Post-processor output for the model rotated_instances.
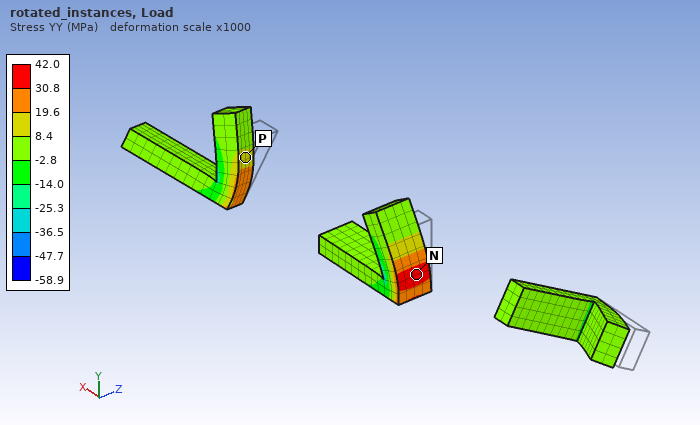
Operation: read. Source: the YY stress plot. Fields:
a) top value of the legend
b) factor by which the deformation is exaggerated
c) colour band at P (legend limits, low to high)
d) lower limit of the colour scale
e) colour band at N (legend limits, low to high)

42.0 MPa
1000
8.4 to 19.6 MPa
-58.9 MPa
30.8 to 42.0 MPa
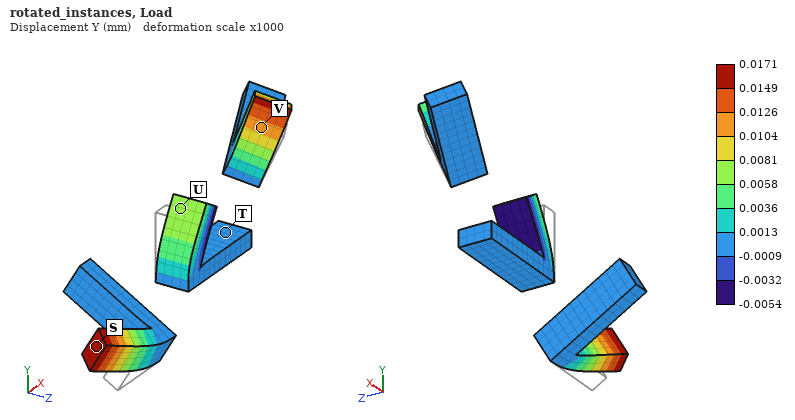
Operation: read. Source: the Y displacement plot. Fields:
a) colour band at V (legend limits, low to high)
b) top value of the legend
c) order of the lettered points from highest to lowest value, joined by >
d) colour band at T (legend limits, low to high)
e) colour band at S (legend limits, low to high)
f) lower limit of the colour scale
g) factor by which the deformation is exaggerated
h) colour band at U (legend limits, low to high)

0.0104 to 0.0126 mm
0.0171 mm
S > V > U > T
-0.0009 to 0.0013 mm
0.0149 to 0.0171 mm
-0.0054 mm
1000
0.0058 to 0.0081 mm
